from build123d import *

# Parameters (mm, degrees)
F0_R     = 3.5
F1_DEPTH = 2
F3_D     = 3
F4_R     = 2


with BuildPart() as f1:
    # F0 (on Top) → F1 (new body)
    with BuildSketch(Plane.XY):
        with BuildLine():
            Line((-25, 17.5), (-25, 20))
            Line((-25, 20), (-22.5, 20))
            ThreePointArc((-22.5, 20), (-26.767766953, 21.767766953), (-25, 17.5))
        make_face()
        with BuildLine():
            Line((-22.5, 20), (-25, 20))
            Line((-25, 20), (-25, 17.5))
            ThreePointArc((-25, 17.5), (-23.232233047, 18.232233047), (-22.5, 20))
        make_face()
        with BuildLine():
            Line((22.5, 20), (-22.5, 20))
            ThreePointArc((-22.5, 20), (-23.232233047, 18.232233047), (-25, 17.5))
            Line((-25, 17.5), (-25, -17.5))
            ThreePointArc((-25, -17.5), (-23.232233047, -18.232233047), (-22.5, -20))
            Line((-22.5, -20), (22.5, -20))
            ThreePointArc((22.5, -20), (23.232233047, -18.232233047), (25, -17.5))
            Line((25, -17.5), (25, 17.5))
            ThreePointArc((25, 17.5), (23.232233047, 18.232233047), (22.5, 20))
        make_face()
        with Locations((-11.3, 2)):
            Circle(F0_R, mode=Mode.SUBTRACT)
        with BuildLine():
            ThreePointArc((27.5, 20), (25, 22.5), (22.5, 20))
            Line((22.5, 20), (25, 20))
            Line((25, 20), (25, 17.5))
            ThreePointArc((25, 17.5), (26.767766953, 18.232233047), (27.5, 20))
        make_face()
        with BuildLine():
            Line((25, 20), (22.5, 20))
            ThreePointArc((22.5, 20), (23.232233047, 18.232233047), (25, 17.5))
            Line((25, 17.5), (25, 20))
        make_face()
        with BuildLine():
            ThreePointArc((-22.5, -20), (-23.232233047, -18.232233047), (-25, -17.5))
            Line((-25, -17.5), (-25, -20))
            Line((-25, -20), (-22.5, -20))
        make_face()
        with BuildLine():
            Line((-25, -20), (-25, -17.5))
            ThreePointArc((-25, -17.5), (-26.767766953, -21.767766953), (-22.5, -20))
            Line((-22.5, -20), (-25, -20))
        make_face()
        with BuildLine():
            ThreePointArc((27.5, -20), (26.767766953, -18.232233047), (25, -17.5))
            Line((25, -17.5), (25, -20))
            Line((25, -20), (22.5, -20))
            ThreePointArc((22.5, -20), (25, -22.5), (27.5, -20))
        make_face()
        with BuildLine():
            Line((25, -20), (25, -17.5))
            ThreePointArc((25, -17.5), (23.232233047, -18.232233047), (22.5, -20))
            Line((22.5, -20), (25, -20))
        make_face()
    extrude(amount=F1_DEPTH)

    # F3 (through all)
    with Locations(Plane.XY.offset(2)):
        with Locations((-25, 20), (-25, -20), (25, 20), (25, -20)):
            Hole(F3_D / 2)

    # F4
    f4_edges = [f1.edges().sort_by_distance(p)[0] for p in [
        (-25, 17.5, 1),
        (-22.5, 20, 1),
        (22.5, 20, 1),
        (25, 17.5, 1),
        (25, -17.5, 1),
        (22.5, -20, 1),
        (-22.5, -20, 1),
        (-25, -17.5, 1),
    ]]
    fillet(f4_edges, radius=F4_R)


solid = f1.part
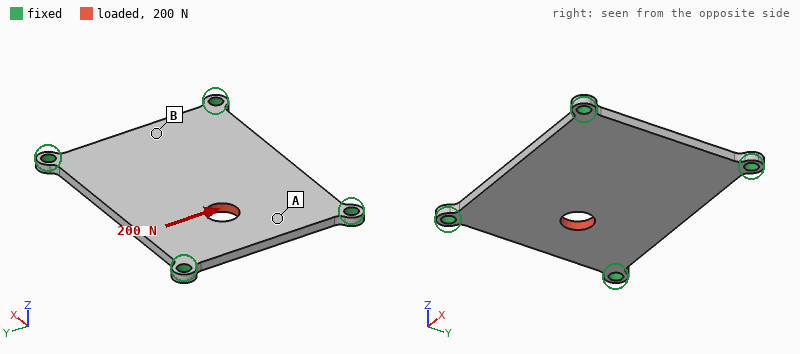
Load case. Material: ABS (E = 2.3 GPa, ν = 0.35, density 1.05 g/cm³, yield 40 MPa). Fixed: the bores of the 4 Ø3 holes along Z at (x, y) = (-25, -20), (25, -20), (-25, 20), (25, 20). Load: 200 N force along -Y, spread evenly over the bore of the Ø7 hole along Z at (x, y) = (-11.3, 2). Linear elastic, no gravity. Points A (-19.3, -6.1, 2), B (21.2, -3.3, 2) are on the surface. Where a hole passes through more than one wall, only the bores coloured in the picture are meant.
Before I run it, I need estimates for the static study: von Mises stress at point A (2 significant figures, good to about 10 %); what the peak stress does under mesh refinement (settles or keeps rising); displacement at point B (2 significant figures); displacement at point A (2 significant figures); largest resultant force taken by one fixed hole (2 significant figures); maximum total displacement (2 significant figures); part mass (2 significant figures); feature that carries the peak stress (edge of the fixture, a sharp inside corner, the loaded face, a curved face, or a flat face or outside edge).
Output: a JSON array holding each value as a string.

["3.4 MPa", "keeps rising", "9.6 µm", "36 µm", "79 N", "60 µm", "4.2 g", "edge of the fixture"]
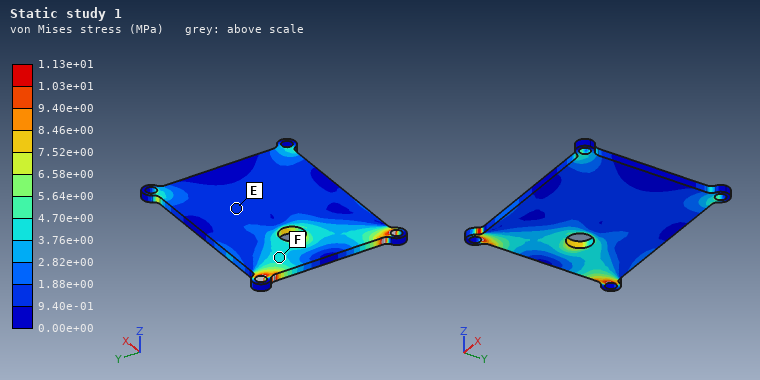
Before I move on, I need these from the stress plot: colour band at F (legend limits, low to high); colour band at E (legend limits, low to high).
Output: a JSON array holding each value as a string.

["3.76e+00 to 4.70e+00 MPa", "9.40e-01 to 1.88e+00 MPa"]
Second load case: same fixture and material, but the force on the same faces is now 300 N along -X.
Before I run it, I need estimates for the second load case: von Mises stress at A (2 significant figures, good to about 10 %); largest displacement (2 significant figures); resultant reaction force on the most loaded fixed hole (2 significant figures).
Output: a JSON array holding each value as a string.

["4.0 MPa", "93 µm", "100 N"]
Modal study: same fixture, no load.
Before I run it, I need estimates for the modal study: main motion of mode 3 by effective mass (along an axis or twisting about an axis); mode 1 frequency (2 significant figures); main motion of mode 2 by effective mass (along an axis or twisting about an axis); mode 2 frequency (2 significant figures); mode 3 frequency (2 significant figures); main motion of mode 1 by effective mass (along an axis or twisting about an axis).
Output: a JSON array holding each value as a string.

["twisting about Y", "850 Hz", "twisting about X", "1500 Hz", "1800 Hz", "along Z"]
